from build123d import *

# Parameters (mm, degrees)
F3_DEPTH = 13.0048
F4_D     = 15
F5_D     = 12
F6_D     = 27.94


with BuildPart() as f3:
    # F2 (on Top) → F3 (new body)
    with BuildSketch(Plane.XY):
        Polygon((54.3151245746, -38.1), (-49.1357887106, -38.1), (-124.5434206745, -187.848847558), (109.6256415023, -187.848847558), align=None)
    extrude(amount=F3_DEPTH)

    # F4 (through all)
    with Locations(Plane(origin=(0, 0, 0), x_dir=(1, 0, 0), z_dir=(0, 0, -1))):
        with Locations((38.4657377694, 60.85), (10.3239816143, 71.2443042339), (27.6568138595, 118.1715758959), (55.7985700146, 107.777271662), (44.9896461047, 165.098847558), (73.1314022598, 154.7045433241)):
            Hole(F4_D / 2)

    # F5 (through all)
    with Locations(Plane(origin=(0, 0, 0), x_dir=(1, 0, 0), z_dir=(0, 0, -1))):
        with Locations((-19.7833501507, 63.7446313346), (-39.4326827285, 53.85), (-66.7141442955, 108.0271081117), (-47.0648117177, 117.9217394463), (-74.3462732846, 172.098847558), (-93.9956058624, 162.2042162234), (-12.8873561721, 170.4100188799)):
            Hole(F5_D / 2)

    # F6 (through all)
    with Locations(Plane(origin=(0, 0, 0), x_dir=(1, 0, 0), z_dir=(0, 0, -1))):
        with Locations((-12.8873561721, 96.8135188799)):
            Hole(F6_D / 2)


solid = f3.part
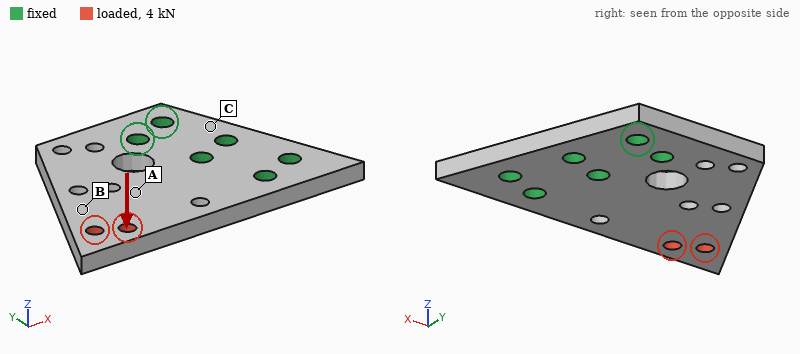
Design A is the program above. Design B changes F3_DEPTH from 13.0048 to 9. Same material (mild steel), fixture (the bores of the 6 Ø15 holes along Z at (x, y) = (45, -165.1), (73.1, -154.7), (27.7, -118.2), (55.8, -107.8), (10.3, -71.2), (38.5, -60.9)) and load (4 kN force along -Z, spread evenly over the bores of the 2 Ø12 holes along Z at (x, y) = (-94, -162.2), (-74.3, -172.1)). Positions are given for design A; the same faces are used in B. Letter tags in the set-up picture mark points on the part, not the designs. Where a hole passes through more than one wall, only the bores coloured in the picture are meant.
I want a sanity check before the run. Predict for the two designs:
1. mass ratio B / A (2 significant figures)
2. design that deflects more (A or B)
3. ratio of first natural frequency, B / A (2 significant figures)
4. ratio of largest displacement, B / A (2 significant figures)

0.69
B
0.70
2.9
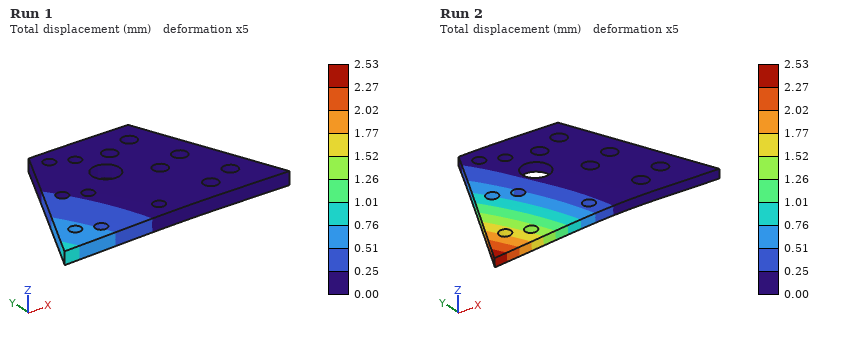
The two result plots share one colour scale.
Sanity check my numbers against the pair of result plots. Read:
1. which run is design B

Run 2
